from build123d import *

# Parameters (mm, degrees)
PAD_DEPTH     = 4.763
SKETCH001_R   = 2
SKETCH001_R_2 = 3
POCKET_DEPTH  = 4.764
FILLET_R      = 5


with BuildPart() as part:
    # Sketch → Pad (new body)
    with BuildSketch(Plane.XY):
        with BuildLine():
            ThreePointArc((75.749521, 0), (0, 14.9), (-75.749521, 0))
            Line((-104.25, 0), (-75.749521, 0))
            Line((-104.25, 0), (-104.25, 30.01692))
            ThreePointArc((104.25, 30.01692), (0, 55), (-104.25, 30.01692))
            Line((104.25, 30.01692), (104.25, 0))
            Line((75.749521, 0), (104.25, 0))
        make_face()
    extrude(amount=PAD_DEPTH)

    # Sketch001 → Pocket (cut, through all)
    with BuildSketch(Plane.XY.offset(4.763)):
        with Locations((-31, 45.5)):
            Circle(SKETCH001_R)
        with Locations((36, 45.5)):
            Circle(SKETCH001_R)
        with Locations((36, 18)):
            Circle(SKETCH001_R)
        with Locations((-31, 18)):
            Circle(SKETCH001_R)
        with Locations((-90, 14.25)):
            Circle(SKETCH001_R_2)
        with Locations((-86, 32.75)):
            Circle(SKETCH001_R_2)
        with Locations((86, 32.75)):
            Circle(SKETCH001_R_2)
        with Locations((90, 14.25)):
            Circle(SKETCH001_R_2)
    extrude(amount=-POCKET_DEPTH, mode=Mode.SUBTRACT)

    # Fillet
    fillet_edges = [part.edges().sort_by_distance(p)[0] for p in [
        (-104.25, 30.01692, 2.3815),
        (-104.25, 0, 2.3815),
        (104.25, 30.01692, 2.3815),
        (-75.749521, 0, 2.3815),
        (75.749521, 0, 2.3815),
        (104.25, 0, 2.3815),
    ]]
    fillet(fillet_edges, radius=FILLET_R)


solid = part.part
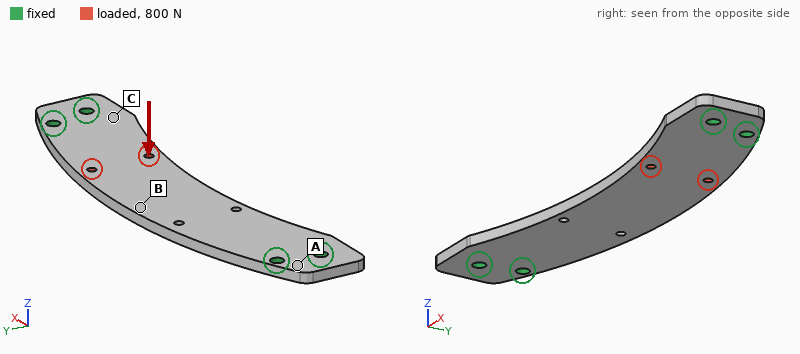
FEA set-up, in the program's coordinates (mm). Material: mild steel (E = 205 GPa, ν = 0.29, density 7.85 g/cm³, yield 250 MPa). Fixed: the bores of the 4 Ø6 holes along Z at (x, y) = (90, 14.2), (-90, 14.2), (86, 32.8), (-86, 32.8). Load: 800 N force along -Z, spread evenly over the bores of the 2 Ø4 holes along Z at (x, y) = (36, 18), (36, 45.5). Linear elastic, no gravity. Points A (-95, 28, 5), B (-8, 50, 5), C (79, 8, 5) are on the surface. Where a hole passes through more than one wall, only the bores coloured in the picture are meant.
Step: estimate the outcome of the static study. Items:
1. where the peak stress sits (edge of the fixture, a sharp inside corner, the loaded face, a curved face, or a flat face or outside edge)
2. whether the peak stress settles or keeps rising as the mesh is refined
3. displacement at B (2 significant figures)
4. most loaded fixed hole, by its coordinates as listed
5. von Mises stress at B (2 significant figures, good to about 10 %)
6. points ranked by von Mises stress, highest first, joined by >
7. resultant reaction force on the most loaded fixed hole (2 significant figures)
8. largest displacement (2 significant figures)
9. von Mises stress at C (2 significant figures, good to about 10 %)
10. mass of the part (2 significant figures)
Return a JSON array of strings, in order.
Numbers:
["edge of the fixture", "keeps rising", "0.18 mm", "(86, 32.8)", "29 MPa", "C > B > A", "660 N", "0.22 mm", "68 MPa", "300 g"]
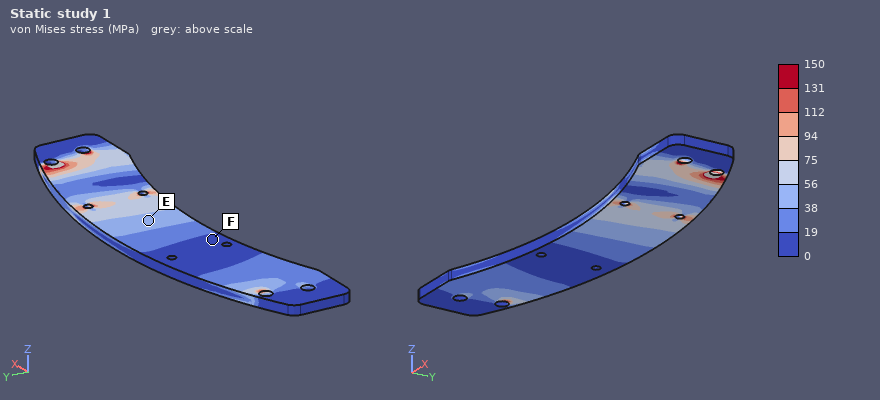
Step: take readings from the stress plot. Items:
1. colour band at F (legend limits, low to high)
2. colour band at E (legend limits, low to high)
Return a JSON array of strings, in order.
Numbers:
["0 to 19 MPa", "38 to 56 MPa"]
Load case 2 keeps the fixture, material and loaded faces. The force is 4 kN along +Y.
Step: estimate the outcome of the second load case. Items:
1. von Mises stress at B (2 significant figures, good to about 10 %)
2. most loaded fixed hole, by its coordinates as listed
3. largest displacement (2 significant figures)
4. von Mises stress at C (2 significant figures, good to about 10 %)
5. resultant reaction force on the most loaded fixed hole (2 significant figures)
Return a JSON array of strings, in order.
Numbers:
["19 MPa", "(90, 14.2)", "27 µm", "34 MPa", "4.3 kN"]
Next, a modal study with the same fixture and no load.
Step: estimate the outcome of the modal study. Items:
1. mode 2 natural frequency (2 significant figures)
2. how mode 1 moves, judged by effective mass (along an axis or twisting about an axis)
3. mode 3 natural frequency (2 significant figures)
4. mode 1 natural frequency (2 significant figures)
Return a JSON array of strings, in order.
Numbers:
["2300 Hz", "along Z", "2300 Hz", "830 Hz"]
